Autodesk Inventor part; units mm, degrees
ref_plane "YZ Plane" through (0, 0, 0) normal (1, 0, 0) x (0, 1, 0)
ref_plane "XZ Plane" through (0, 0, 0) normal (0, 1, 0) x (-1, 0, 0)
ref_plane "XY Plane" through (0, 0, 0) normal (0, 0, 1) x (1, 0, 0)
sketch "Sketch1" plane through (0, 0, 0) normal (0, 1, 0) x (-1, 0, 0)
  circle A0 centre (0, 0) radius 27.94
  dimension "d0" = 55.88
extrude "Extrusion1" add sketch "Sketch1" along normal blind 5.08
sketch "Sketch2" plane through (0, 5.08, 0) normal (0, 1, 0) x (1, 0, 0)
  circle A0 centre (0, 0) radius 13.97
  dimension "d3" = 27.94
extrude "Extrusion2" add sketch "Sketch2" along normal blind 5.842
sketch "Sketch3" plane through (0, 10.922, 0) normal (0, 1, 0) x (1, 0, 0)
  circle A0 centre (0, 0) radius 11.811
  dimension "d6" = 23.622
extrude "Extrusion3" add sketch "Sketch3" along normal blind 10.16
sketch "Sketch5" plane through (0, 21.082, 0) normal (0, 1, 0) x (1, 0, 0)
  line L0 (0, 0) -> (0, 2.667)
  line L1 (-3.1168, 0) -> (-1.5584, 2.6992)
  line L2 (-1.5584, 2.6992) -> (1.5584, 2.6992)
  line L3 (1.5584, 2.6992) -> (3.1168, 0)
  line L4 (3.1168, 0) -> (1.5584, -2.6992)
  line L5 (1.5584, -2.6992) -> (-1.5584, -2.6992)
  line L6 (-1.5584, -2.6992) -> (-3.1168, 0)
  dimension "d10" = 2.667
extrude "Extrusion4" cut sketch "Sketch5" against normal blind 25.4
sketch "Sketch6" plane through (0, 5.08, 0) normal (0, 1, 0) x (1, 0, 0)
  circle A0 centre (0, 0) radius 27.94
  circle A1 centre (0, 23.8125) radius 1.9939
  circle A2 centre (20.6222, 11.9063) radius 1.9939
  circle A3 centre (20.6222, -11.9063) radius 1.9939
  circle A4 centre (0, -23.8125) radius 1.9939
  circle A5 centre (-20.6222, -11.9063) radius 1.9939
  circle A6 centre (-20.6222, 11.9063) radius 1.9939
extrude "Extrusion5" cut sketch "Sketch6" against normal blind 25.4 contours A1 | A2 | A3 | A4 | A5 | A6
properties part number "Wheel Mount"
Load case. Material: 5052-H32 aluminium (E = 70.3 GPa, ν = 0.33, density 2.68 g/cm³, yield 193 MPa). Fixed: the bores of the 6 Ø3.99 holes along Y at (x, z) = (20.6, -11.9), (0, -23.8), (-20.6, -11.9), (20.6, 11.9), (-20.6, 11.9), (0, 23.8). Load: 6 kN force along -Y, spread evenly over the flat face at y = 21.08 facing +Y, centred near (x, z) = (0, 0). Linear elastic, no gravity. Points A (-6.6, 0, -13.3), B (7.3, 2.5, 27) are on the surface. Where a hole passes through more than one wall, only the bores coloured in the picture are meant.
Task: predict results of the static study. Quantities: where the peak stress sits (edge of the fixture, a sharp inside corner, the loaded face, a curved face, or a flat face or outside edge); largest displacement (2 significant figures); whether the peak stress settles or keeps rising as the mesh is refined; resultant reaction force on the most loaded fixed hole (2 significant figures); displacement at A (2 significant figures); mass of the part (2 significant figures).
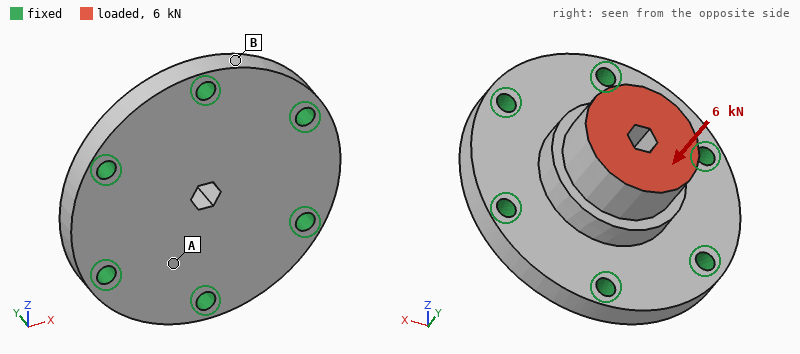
edge of the fixture
22 µm
keeps rising
1.1 kN
15 µm
52 g
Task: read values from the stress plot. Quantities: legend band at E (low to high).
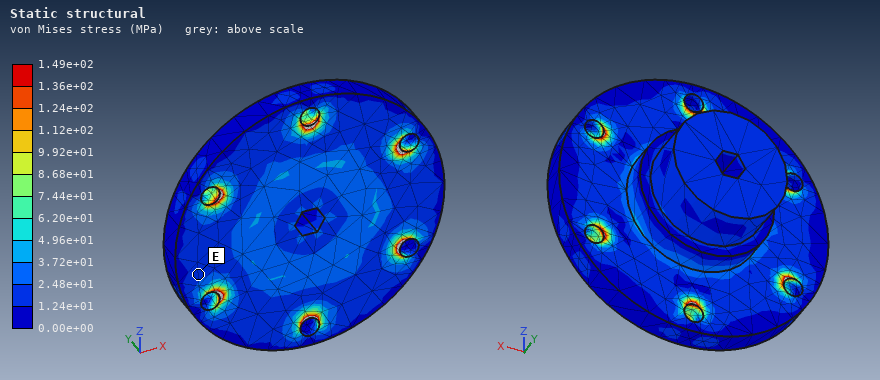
1.24e+01 to 2.48e+01 MPa
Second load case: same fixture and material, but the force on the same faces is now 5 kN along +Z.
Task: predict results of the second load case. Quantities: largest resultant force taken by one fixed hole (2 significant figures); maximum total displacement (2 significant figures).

2.0 kN
48 µm
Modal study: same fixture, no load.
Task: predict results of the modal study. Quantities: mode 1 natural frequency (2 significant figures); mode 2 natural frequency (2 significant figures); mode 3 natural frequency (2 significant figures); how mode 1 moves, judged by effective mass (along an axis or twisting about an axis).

16 kHz
18 kHz
18 kHz
along Y
